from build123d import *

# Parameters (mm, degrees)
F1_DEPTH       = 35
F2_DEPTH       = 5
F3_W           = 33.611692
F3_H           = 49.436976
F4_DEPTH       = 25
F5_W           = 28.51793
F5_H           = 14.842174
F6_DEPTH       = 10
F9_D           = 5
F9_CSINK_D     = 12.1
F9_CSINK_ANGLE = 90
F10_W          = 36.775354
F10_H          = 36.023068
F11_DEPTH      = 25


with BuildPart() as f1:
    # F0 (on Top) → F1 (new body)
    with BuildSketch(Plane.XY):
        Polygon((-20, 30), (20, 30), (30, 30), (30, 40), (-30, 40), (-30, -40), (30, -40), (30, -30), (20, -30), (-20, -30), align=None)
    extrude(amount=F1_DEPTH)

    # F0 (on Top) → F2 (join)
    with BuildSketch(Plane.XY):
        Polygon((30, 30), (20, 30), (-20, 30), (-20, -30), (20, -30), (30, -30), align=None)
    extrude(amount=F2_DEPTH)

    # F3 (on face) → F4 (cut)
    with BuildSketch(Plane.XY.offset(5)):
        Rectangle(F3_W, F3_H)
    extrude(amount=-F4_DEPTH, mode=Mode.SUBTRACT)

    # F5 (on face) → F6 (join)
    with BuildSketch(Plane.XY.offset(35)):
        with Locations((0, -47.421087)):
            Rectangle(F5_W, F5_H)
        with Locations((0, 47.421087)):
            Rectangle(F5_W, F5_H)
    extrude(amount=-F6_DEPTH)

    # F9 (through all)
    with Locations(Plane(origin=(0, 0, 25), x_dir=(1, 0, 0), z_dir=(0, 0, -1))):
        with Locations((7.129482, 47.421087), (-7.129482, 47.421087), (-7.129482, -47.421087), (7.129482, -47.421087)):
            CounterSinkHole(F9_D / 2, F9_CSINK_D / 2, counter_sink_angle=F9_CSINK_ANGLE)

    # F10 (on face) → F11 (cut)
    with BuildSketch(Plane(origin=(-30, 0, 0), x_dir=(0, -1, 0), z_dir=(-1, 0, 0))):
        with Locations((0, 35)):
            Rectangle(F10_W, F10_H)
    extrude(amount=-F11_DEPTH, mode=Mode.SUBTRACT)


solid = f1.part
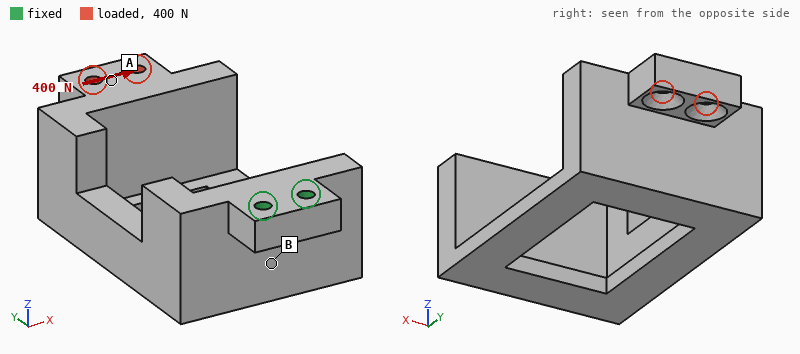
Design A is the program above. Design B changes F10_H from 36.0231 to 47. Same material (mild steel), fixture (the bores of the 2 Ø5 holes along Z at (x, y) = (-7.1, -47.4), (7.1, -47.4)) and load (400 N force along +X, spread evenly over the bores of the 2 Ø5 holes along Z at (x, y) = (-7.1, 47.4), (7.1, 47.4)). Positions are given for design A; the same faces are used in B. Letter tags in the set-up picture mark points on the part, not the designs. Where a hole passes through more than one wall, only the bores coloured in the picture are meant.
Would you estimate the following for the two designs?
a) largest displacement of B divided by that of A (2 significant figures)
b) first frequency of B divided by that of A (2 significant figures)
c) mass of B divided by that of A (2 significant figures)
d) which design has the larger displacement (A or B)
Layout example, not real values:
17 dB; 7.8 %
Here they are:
1.2; 0.87; 0.97; B
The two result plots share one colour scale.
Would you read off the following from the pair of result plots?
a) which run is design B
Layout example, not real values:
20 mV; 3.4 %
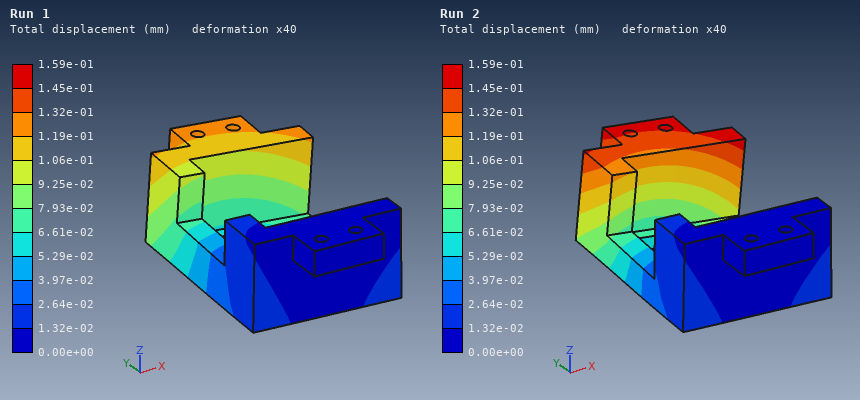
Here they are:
Run 2
